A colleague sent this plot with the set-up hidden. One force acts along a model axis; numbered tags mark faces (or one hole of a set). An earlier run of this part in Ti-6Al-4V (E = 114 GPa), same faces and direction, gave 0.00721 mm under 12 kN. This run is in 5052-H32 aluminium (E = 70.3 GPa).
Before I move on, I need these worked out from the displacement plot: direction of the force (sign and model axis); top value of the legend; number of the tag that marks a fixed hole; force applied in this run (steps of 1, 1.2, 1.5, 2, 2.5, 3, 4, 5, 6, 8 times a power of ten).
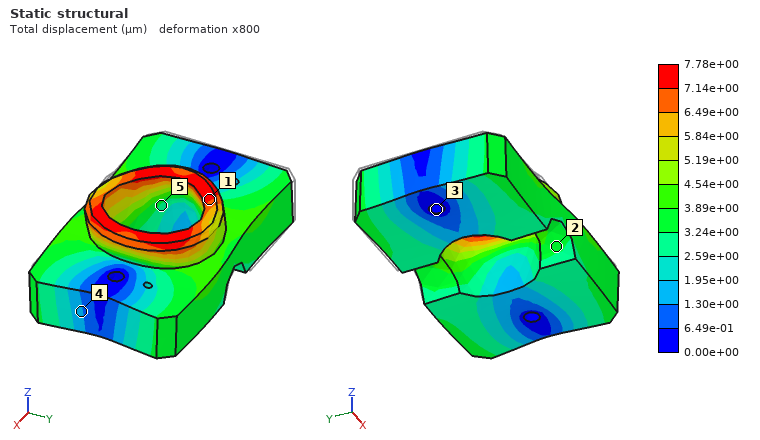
+X
7.78e+00 µm
3
8 kN
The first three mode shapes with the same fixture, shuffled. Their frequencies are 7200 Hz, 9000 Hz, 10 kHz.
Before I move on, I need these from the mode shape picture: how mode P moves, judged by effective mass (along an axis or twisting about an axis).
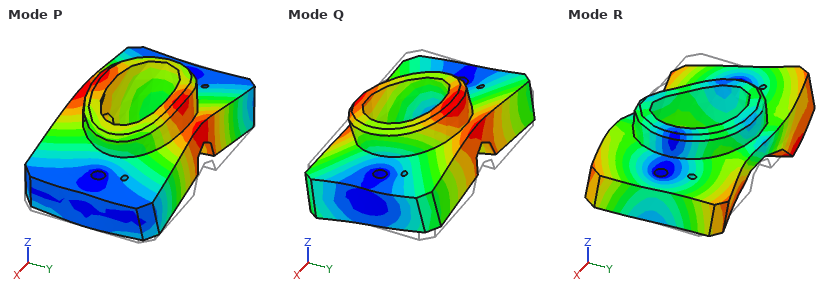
along Z
